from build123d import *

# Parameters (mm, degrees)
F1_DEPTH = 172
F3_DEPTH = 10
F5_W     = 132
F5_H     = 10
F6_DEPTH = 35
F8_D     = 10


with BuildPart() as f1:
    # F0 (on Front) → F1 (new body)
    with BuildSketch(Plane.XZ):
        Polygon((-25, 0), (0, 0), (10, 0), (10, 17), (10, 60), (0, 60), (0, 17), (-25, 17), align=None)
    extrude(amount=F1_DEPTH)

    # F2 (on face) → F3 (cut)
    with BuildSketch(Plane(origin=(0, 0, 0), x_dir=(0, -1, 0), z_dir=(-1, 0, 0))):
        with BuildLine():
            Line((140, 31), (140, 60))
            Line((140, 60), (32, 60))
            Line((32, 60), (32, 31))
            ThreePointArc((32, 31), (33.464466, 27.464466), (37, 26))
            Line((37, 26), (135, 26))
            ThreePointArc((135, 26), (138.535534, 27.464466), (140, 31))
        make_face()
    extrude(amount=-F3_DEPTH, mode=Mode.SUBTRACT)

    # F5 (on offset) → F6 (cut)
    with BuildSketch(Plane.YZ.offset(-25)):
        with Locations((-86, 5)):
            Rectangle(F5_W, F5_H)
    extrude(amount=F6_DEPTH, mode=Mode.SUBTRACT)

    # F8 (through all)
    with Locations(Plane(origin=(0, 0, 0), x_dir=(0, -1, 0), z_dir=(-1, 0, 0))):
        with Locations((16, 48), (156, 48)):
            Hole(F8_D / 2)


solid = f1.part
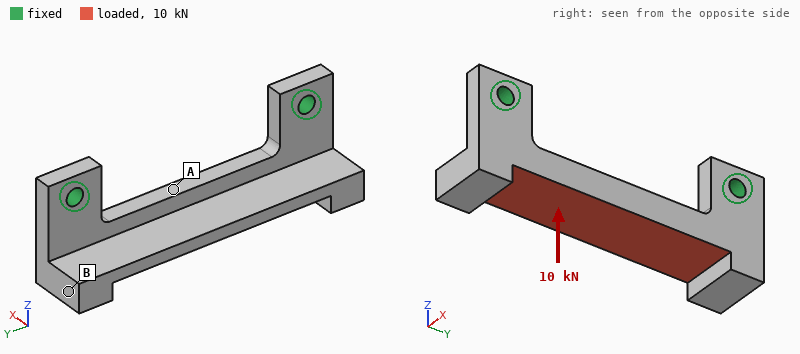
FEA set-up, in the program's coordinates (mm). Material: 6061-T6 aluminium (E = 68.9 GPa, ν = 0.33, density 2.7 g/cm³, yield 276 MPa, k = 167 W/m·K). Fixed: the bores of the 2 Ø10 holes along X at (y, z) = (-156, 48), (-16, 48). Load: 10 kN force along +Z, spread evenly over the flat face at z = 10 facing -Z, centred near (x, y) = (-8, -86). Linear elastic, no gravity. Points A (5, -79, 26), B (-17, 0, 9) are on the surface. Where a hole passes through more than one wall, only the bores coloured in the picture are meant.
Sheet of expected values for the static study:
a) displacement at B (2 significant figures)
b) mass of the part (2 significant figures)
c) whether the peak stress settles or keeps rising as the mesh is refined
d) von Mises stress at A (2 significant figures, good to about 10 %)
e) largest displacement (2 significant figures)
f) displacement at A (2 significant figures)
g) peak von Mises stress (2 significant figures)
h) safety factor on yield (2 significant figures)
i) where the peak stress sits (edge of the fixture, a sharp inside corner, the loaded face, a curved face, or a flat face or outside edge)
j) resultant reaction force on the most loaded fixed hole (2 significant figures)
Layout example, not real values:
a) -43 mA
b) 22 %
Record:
a) 0.28 mm
b) 250 g
c) settles
d) 64 MPa
e) 0.78 mm
f) 0.18 mm
g) 390 MPa
h) 0.71
i) a curved face
j) 6.2 kN
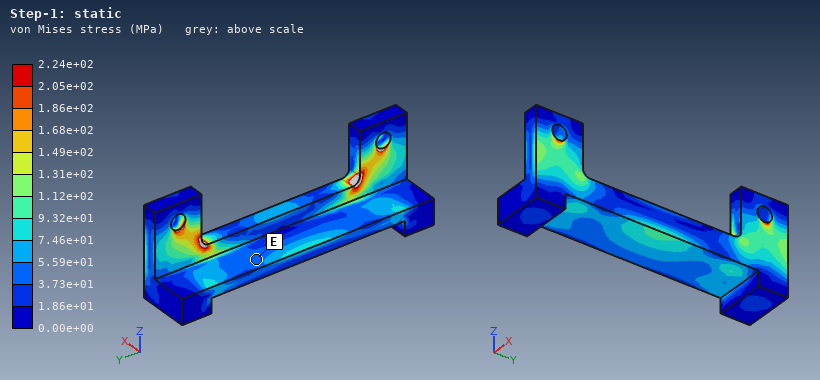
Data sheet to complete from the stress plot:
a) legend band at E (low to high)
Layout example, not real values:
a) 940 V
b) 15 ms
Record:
a) 3.73e+01 to 5.59e+01 MPa
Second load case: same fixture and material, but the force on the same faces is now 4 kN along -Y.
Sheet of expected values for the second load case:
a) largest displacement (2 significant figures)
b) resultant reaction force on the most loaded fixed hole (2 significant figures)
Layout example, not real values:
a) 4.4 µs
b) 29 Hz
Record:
a) 49 µm
b) 2.1 kN
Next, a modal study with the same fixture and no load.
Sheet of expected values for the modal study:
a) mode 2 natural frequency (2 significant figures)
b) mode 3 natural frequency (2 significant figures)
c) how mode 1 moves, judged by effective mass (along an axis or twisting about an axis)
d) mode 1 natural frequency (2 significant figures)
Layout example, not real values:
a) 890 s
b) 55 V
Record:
a) 2300 Hz
b) 3400 Hz
c) along X
d) 1600 Hz
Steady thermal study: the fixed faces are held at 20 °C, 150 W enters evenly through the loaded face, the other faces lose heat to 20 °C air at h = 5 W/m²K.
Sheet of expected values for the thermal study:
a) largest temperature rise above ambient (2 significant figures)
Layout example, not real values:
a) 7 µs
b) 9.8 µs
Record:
a) 82 K
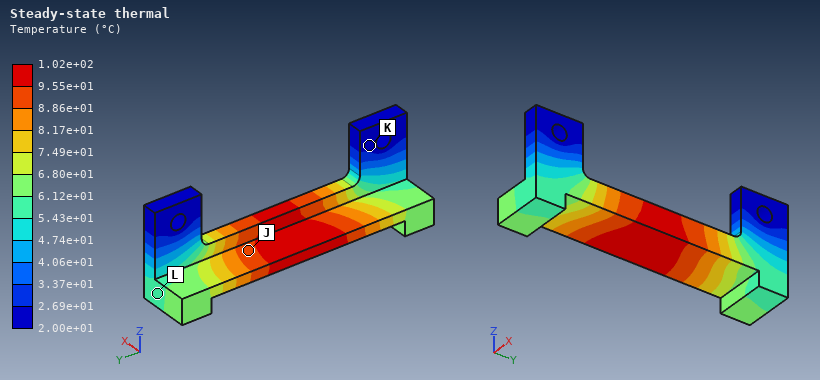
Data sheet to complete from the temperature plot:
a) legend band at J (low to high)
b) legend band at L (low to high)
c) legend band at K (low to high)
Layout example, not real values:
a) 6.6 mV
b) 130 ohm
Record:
a) 8.86e+01 to 9.55e+01 °C
b) 5.43e+01 to 6.12e+01 °C
c) 2.00e+01 to 2.69e+01 °C
